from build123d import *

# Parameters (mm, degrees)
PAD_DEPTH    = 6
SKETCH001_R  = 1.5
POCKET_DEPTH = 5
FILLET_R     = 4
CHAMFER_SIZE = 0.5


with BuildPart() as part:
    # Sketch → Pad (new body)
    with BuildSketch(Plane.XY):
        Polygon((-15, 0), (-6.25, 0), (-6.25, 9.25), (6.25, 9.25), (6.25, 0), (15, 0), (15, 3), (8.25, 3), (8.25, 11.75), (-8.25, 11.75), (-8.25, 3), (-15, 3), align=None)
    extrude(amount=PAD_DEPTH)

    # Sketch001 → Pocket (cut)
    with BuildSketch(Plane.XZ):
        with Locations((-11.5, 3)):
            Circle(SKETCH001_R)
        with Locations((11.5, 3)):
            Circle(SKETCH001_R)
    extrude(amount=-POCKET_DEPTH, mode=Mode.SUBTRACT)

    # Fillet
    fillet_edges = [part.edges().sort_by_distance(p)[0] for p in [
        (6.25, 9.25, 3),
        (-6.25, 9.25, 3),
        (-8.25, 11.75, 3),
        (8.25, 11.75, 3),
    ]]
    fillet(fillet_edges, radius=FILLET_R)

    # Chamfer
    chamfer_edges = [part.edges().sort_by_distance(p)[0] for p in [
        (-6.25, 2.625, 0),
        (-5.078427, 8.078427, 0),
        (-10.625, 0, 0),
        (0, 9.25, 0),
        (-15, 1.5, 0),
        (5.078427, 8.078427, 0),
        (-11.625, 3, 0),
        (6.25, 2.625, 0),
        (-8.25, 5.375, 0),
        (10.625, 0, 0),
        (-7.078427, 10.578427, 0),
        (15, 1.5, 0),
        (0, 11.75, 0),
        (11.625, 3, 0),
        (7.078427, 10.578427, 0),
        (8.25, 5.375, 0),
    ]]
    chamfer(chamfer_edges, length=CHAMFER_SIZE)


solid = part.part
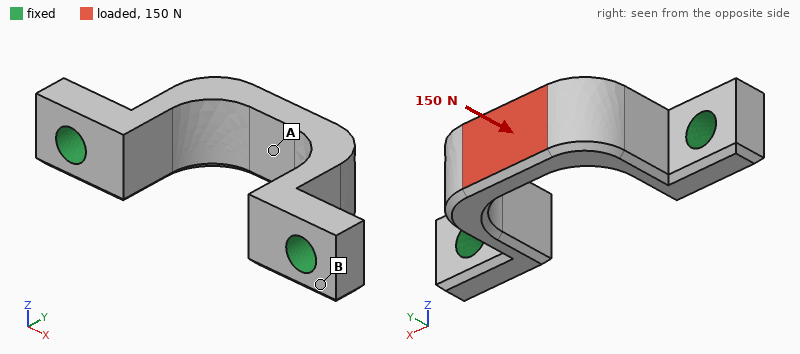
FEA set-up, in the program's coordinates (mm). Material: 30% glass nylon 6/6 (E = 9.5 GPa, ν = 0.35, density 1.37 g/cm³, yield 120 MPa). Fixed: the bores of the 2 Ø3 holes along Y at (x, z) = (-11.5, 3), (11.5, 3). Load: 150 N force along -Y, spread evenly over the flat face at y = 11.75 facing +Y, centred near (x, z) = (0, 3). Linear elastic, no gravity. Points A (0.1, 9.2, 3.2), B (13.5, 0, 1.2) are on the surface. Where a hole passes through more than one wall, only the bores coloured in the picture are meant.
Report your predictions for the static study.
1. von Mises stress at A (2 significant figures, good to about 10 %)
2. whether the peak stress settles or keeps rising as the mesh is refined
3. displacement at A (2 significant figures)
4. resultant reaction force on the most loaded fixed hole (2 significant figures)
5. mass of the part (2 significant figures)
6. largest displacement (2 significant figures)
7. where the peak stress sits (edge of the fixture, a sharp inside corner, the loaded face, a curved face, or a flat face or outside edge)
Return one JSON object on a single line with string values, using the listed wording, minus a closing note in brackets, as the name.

{"von Mises stress at A": "17 MPa", "whether the peak stress settles or keeps rising as the mesh is refined": "keeps rising", "displacement at A": "34 µm", "resultant reaction force on the most loaded fixed hole": "87 N", "mass of the part": "0.90 g", "largest displacement": "40 µm", "where the peak stress sits": "edge of the fixture"}
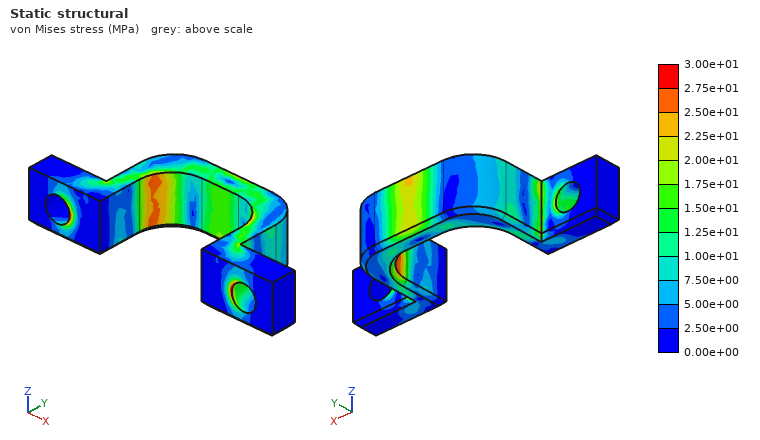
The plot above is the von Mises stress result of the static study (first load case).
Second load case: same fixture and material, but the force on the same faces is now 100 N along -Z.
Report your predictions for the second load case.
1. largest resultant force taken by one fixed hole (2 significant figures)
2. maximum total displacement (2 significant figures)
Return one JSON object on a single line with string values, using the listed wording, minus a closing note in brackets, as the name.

{"largest resultant force taken by one fixed hole": "50 N", "maximum total displacement": "0.18 mm"}
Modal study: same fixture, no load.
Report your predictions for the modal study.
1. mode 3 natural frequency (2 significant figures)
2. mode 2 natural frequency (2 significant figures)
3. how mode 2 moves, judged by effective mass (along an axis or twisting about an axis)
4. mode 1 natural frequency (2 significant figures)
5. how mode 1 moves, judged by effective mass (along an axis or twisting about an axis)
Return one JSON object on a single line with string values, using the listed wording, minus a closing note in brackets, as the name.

{"mode 3 natural frequency": "14 kHz", "mode 2 natural frequency": "11 kHz", "how mode 2 moves, judged by effective mass": "along X", "mode 1 natural frequency": "7300 Hz", "how mode 1 moves, judged by effective mass": "along Z"}
